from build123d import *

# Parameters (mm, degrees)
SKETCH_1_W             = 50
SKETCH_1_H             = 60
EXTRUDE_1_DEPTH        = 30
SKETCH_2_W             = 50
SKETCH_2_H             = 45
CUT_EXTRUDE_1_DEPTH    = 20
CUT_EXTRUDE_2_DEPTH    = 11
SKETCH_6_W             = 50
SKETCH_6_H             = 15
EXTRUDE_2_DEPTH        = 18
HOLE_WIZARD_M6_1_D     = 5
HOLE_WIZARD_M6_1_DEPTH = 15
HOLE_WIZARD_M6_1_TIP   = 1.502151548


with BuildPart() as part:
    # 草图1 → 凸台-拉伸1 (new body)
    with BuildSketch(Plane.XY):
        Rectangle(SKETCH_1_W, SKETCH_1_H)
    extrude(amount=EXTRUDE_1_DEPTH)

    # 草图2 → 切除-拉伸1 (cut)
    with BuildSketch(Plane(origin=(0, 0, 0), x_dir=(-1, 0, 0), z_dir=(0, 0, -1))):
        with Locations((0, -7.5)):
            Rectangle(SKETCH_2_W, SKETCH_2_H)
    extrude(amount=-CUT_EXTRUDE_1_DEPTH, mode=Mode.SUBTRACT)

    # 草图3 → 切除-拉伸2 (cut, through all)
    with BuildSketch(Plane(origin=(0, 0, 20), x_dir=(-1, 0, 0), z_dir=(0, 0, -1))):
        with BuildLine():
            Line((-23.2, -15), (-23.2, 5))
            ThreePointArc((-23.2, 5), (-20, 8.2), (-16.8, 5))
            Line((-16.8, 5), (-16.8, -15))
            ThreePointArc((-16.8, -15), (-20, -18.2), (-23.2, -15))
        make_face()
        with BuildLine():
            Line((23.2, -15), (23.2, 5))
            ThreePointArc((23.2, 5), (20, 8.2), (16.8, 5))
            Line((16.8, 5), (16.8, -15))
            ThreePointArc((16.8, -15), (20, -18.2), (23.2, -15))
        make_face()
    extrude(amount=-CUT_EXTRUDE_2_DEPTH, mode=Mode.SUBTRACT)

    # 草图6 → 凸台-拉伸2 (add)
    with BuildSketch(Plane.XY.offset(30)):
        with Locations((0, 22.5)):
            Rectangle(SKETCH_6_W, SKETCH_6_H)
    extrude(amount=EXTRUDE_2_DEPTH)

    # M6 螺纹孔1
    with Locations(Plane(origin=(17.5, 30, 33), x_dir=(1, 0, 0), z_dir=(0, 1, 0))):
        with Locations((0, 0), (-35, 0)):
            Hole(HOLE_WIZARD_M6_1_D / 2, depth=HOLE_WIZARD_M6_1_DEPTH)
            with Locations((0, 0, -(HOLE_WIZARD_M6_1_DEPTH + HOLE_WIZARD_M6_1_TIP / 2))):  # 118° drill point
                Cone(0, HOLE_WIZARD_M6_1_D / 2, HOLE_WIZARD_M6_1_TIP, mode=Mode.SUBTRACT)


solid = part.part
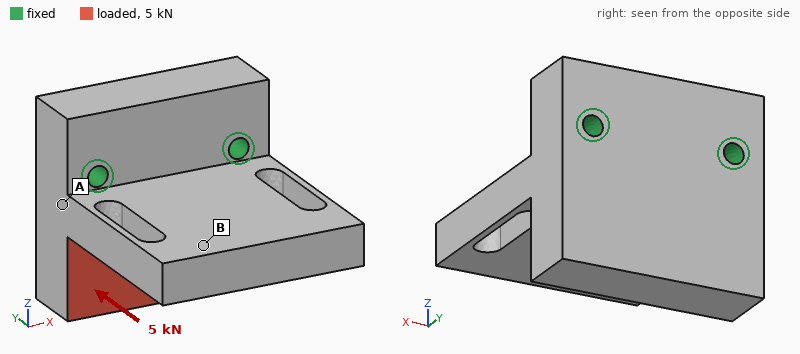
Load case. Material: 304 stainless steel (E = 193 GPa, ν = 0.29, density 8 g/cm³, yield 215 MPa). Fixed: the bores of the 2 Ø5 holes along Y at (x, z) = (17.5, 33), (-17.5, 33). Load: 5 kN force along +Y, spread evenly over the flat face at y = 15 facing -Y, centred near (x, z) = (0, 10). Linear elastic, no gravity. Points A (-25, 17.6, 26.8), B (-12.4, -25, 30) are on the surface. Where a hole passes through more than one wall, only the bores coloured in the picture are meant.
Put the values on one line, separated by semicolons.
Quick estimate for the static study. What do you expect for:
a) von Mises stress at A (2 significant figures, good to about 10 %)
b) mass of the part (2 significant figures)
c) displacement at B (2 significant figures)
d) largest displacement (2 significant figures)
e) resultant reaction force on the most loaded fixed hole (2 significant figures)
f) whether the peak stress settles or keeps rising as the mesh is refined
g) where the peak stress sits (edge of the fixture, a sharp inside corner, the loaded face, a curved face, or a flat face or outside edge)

30 MPa; 440 g; 21 µm; 24 µm; 2.5 kN; keeps rising; edge of the fixture
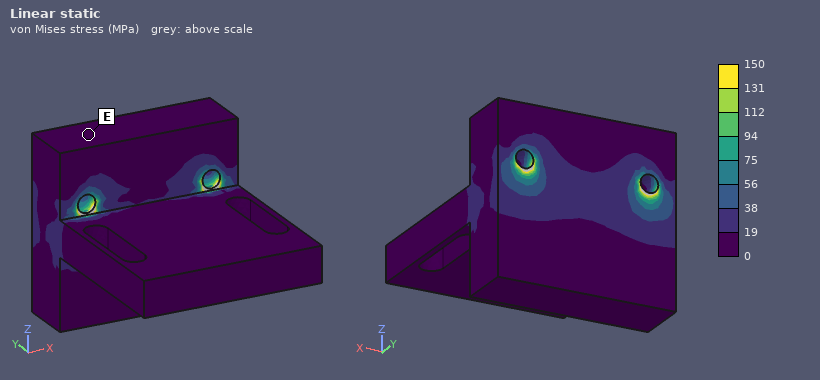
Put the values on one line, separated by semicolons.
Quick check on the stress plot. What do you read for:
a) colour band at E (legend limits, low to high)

0 to 19 MPa
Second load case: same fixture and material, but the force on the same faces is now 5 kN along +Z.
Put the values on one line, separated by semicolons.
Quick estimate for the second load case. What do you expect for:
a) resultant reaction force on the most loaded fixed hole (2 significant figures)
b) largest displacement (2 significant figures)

2.5 kN; 8.2 µm
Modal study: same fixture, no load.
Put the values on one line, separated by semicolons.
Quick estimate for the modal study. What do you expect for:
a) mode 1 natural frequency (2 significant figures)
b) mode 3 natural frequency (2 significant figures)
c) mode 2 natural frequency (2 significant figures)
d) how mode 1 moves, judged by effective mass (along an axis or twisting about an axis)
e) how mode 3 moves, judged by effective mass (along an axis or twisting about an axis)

2900 Hz; 7900 Hz; 6700 Hz; along Z; along X
